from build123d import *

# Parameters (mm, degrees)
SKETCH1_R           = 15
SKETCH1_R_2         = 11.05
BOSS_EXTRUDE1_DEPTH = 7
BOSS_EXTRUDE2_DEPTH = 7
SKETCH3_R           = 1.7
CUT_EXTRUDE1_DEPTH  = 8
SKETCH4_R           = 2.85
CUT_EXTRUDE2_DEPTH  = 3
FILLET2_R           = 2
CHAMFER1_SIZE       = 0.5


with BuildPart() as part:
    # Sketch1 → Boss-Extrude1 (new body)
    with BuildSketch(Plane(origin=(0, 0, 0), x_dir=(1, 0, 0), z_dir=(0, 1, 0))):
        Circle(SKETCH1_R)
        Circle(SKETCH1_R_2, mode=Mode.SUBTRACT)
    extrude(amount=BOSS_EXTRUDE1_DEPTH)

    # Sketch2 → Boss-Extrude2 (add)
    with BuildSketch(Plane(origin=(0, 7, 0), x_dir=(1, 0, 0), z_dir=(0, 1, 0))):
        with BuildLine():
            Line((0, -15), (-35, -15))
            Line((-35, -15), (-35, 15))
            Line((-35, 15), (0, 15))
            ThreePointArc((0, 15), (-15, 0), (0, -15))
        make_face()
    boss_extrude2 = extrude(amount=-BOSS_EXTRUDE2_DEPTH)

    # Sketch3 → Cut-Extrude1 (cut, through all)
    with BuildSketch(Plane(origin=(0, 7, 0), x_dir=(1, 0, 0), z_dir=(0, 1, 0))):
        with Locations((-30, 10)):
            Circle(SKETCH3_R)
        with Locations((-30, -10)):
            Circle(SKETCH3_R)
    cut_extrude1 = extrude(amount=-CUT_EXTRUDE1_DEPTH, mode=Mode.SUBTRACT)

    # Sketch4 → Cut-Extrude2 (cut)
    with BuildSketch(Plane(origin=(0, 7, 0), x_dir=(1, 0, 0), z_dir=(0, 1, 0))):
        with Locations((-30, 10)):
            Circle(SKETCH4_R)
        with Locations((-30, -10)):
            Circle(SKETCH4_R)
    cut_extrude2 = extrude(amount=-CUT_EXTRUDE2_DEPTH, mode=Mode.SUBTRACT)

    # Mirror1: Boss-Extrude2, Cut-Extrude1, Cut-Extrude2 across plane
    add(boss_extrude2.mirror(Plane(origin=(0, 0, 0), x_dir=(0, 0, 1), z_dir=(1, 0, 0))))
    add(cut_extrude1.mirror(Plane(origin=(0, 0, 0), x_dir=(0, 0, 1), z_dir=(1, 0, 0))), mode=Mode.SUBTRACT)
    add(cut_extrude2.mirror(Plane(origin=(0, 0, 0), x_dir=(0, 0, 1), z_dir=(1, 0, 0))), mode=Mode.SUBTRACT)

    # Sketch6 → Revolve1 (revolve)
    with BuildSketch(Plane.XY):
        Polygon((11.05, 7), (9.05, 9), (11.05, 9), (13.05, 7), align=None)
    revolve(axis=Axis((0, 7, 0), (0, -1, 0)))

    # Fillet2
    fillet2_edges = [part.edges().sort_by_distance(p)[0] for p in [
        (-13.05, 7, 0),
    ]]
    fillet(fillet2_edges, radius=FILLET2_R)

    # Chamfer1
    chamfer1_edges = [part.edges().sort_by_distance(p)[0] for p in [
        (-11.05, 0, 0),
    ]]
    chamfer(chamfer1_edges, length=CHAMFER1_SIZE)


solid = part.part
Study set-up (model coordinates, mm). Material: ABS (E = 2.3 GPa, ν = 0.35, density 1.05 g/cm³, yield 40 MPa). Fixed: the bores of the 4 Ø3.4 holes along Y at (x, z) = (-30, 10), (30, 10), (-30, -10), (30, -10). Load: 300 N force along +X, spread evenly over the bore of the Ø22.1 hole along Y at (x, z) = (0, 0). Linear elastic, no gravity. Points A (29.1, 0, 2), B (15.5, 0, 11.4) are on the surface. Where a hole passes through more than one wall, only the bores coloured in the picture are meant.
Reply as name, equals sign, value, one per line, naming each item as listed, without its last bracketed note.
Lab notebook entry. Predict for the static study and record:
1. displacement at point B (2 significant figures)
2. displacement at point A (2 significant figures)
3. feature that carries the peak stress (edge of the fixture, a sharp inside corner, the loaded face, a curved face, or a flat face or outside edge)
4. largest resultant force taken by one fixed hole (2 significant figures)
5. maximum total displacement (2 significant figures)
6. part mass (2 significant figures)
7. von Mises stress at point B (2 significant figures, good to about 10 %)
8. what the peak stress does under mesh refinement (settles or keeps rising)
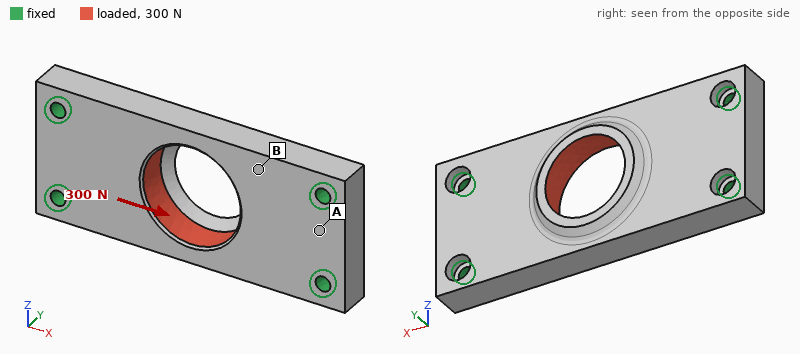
displacement at point B = 8.1 µm
displacement at point A = 3.5 µm
feature that carries the peak stress = edge of the fixture
largest resultant force taken by one fixed hole = 76 N
maximum total displacement = 13 µm
part mass = 12 g
von Mises stress at point B = 1.1 MPa
what the peak stress does under mesh refinement = keeps rising
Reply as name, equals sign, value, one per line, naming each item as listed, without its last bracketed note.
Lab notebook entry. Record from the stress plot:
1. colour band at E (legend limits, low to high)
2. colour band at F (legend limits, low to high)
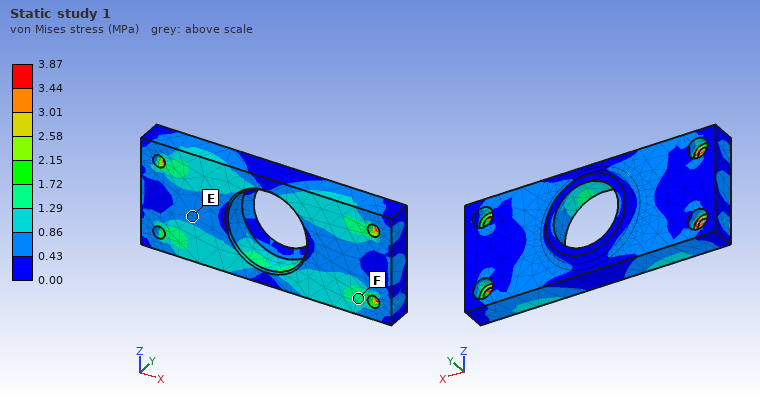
colour band at E = 0.43 to 0.86 MPa
colour band at F = 1.29 to 1.72 MPa
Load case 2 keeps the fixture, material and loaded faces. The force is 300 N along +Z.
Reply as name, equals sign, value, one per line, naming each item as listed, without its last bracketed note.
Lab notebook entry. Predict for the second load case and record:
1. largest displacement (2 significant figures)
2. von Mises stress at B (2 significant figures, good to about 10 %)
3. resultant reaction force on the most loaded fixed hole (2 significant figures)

largest displacement = 48 µm
von Mises stress at B = 0.66 MPa
resultant reaction force on the most loaded fixed hole = 110 N
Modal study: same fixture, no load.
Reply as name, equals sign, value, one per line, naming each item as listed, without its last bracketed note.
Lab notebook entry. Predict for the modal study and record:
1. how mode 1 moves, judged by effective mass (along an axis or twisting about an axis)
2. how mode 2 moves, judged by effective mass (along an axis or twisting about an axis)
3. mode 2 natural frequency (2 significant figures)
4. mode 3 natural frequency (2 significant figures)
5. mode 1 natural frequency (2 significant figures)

how mode 1 moves, judged by effective mass = along Y
how mode 2 moves, judged by effective mass = twisting about X
mode 2 natural frequency = 3800 Hz
mode 3 natural frequency = 5100 Hz
mode 1 natural frequency = 2400 Hz
